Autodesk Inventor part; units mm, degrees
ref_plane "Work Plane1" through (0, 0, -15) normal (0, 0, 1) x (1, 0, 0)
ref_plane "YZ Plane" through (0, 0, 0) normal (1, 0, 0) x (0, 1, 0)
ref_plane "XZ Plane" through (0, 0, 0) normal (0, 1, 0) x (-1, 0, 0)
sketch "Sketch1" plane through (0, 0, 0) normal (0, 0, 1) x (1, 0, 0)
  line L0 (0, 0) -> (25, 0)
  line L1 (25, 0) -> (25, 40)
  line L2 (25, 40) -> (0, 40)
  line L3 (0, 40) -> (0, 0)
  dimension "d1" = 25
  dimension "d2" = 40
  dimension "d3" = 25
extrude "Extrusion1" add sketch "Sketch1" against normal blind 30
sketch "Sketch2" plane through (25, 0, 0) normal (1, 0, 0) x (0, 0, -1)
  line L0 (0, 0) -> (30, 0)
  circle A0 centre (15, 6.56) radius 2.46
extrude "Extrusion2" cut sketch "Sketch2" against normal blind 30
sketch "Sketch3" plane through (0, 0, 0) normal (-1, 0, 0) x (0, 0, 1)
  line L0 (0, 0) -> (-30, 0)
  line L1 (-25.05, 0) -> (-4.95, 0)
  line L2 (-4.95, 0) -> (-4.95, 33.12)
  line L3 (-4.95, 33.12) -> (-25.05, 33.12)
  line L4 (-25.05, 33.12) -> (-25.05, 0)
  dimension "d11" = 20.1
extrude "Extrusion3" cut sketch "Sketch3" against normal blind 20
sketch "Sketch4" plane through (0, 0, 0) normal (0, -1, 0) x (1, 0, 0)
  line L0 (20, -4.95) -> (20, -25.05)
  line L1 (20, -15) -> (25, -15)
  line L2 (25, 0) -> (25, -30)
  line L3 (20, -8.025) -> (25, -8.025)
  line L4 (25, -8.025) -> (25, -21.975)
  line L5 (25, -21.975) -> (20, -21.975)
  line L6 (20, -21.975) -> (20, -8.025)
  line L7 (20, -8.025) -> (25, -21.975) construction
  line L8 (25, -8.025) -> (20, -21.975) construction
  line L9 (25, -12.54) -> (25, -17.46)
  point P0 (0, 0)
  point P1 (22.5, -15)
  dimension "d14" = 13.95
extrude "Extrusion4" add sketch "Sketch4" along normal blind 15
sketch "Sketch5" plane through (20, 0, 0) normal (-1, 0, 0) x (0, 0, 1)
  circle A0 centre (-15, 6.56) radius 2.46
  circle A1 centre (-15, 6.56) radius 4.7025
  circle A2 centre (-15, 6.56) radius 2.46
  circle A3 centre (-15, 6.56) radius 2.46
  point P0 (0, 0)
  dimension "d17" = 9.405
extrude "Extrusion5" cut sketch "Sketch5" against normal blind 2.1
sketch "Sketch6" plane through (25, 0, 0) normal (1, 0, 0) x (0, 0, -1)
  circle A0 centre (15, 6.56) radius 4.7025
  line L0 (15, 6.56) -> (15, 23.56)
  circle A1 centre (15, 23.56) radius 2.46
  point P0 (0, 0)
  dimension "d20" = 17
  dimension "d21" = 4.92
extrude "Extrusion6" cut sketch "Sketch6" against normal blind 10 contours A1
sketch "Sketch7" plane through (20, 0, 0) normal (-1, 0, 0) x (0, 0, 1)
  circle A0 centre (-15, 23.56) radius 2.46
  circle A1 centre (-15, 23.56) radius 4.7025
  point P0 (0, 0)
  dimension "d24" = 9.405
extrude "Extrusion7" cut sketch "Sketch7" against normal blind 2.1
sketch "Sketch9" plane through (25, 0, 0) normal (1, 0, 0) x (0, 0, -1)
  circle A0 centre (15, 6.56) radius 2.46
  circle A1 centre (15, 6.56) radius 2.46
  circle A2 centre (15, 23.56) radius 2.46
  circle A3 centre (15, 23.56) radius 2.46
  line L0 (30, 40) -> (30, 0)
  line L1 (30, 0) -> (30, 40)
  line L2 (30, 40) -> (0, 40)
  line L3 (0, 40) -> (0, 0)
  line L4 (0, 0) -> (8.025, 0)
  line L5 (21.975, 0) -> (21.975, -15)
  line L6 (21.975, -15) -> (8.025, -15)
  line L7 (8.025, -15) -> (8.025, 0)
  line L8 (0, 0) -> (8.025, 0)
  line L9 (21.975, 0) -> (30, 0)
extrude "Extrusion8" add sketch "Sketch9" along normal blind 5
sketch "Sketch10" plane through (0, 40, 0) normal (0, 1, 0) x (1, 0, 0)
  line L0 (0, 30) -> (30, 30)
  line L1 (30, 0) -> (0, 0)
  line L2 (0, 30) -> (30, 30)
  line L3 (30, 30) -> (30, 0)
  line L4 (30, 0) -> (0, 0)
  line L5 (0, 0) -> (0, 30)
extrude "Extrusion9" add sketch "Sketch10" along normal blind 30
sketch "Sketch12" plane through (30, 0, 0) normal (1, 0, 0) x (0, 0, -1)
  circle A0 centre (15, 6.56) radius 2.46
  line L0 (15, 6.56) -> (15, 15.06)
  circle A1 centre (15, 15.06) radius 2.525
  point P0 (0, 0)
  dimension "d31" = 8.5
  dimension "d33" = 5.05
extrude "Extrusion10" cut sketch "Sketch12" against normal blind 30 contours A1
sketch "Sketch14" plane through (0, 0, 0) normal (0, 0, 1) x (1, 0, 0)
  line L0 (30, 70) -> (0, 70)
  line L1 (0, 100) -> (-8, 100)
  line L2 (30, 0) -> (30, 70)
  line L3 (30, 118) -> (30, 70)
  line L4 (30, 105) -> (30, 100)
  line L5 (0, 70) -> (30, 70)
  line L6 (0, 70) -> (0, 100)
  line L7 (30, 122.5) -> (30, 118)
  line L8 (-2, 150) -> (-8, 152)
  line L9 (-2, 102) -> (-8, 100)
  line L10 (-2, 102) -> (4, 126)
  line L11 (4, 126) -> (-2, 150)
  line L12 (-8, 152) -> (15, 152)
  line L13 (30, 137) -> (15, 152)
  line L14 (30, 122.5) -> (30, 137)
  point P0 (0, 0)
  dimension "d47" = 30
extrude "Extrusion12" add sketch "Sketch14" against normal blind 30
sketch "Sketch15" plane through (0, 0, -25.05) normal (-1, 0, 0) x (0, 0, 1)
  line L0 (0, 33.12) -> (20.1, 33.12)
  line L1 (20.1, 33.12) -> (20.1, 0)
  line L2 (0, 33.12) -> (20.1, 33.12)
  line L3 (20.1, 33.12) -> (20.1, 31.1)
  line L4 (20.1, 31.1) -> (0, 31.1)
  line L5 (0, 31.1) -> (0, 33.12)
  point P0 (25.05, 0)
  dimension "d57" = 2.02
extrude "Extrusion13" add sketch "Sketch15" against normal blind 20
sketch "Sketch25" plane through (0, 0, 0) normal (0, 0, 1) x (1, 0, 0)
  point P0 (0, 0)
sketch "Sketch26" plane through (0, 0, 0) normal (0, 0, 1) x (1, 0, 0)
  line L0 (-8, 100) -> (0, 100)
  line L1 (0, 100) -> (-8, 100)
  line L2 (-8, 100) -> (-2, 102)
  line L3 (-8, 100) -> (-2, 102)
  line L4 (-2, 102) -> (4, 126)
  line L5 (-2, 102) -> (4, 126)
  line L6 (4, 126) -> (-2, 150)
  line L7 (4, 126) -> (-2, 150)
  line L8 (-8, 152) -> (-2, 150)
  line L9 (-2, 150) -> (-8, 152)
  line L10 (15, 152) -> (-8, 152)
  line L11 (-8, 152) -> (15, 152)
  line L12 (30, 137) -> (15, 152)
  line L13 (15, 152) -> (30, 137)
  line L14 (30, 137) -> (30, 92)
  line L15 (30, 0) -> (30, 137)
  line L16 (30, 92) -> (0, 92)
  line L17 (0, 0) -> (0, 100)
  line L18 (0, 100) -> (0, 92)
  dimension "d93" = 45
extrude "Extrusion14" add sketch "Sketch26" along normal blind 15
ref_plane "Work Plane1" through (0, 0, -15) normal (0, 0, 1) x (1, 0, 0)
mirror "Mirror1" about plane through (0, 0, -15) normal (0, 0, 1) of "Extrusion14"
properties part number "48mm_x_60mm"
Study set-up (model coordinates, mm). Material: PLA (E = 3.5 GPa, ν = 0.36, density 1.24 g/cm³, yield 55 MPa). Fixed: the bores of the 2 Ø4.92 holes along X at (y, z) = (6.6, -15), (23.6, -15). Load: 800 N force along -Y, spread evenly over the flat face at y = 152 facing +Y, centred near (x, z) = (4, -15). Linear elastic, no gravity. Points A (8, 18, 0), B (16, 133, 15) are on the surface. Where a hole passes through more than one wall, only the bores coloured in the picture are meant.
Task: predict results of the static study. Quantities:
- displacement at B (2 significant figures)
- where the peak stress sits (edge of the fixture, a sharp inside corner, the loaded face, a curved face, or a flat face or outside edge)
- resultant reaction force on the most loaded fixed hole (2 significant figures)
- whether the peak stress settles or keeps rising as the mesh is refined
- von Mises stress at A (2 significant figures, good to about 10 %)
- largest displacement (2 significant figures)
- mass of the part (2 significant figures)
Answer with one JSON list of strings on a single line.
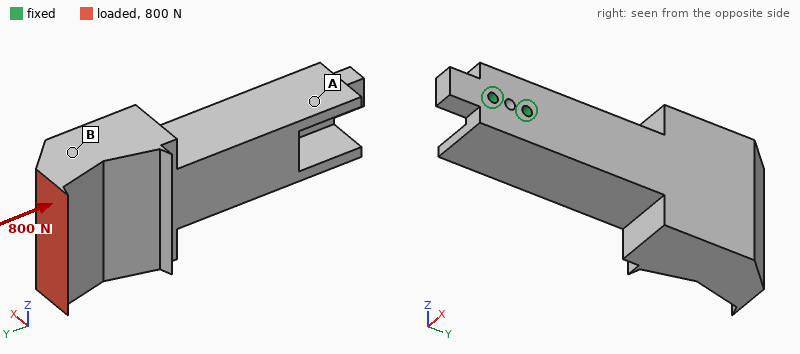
["1.0 mm", "edge of the fixture", "830 N", "keeps rising", "4.4 MPa", "1.4 mm", "210 g"]
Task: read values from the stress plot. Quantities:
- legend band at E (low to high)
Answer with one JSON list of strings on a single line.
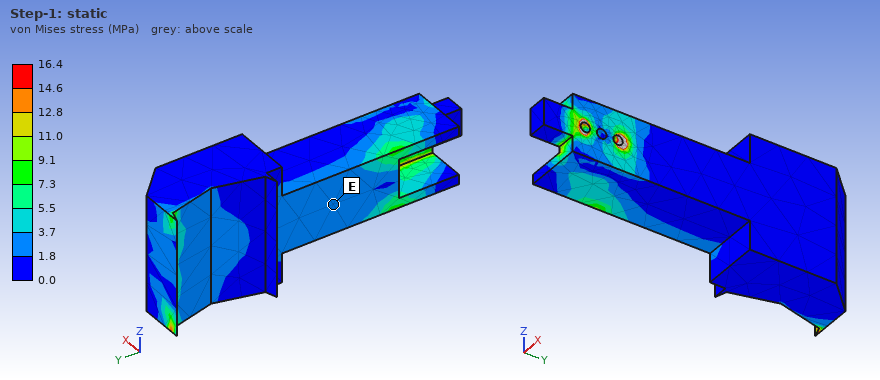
["1.8 to 3.7 MPa"]
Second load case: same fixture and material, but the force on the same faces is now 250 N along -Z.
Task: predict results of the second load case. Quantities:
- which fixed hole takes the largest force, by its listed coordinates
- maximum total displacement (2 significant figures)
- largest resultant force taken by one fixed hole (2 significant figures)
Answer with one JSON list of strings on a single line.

["(23.6, -15)", "2.0 mm", "1.6 kN"]
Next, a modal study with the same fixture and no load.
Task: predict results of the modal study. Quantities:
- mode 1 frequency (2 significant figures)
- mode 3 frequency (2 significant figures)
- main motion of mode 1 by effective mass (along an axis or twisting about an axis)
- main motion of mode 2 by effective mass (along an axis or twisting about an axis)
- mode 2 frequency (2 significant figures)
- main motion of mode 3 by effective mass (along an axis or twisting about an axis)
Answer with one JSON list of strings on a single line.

["190 Hz", "570 Hz", "along X", "along Z", "210 Hz", "twisting about Y"]
